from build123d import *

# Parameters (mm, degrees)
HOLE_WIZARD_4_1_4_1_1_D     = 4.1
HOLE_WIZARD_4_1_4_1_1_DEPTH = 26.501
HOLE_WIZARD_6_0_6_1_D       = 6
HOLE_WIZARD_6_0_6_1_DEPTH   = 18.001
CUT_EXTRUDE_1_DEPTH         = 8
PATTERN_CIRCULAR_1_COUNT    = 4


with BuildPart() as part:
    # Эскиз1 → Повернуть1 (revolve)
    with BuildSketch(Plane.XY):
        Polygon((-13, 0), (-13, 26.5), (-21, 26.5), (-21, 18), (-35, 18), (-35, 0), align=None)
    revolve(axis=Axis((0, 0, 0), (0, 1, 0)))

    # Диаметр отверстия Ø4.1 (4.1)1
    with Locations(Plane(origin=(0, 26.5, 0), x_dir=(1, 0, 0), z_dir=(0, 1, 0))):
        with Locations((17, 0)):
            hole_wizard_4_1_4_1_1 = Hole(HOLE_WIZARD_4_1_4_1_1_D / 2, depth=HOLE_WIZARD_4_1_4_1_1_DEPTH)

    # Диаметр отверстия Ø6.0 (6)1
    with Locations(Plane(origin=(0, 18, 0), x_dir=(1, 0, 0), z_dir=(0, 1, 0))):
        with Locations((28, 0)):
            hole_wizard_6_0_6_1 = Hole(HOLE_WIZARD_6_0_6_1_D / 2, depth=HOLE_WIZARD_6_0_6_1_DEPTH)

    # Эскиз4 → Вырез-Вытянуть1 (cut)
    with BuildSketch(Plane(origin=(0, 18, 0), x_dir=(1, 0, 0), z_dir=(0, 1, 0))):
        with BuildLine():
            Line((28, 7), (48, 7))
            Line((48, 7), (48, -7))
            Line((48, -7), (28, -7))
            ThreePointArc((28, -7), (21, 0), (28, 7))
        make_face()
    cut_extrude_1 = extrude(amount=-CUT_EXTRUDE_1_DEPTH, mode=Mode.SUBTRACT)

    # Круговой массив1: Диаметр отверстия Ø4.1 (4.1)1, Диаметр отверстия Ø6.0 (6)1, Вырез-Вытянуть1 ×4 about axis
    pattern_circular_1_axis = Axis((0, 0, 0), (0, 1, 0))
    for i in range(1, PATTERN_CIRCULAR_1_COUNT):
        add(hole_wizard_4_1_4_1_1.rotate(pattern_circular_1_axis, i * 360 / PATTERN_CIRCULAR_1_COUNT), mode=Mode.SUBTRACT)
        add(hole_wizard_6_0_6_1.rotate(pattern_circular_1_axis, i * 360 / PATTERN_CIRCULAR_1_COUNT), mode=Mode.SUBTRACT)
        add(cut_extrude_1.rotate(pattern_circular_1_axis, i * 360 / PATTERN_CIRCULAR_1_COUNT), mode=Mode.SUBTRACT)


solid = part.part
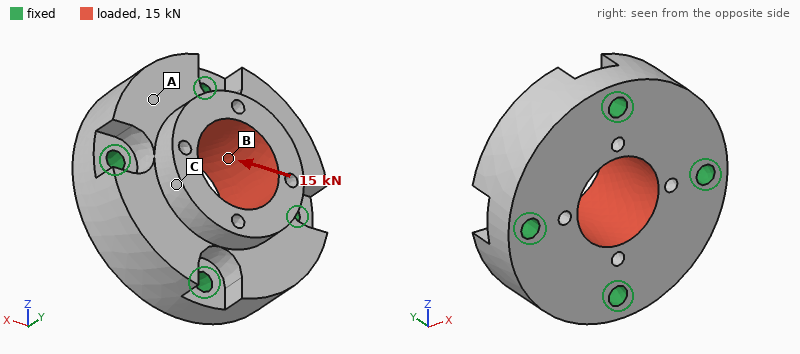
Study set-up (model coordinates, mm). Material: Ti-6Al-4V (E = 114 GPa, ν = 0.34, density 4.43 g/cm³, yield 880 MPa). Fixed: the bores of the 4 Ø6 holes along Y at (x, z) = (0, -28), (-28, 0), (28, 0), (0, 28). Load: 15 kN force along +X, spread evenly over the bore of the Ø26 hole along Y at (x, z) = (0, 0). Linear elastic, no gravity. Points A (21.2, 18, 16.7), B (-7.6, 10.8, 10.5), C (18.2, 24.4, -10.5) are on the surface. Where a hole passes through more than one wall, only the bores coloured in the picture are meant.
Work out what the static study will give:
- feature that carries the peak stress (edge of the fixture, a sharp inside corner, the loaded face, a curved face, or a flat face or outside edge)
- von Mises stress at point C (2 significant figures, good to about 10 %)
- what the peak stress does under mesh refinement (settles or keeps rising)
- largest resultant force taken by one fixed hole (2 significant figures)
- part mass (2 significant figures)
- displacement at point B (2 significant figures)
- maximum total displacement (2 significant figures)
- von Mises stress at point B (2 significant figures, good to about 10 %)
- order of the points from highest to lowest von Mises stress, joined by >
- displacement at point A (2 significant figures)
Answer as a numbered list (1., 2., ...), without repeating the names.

1. edge of the fixture
2. 10 MPa
3. keeps rising
4. 4.7 kN
5. 260 g
6. 4.1 µm
7. 9.1 µm
8. 18 MPa
9. B > C > A
10. 4.7 µm
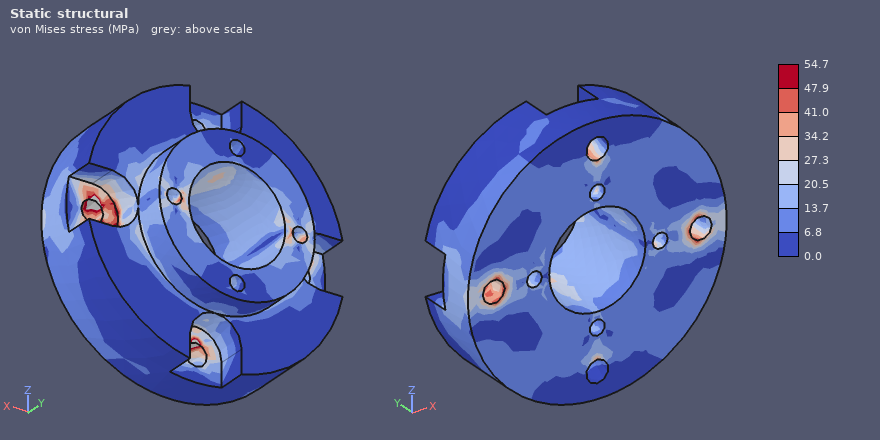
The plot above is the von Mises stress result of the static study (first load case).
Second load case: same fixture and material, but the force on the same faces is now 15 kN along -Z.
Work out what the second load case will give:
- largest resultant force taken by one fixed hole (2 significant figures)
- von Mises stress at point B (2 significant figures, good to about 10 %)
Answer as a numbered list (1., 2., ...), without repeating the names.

1. 4.7 kN
2. 17 MPa
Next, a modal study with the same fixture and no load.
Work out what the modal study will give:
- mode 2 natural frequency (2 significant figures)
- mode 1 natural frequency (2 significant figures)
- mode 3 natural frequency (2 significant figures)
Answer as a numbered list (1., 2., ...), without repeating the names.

1. 19 kHz
2. 17 kHz
3. 19 kHz
